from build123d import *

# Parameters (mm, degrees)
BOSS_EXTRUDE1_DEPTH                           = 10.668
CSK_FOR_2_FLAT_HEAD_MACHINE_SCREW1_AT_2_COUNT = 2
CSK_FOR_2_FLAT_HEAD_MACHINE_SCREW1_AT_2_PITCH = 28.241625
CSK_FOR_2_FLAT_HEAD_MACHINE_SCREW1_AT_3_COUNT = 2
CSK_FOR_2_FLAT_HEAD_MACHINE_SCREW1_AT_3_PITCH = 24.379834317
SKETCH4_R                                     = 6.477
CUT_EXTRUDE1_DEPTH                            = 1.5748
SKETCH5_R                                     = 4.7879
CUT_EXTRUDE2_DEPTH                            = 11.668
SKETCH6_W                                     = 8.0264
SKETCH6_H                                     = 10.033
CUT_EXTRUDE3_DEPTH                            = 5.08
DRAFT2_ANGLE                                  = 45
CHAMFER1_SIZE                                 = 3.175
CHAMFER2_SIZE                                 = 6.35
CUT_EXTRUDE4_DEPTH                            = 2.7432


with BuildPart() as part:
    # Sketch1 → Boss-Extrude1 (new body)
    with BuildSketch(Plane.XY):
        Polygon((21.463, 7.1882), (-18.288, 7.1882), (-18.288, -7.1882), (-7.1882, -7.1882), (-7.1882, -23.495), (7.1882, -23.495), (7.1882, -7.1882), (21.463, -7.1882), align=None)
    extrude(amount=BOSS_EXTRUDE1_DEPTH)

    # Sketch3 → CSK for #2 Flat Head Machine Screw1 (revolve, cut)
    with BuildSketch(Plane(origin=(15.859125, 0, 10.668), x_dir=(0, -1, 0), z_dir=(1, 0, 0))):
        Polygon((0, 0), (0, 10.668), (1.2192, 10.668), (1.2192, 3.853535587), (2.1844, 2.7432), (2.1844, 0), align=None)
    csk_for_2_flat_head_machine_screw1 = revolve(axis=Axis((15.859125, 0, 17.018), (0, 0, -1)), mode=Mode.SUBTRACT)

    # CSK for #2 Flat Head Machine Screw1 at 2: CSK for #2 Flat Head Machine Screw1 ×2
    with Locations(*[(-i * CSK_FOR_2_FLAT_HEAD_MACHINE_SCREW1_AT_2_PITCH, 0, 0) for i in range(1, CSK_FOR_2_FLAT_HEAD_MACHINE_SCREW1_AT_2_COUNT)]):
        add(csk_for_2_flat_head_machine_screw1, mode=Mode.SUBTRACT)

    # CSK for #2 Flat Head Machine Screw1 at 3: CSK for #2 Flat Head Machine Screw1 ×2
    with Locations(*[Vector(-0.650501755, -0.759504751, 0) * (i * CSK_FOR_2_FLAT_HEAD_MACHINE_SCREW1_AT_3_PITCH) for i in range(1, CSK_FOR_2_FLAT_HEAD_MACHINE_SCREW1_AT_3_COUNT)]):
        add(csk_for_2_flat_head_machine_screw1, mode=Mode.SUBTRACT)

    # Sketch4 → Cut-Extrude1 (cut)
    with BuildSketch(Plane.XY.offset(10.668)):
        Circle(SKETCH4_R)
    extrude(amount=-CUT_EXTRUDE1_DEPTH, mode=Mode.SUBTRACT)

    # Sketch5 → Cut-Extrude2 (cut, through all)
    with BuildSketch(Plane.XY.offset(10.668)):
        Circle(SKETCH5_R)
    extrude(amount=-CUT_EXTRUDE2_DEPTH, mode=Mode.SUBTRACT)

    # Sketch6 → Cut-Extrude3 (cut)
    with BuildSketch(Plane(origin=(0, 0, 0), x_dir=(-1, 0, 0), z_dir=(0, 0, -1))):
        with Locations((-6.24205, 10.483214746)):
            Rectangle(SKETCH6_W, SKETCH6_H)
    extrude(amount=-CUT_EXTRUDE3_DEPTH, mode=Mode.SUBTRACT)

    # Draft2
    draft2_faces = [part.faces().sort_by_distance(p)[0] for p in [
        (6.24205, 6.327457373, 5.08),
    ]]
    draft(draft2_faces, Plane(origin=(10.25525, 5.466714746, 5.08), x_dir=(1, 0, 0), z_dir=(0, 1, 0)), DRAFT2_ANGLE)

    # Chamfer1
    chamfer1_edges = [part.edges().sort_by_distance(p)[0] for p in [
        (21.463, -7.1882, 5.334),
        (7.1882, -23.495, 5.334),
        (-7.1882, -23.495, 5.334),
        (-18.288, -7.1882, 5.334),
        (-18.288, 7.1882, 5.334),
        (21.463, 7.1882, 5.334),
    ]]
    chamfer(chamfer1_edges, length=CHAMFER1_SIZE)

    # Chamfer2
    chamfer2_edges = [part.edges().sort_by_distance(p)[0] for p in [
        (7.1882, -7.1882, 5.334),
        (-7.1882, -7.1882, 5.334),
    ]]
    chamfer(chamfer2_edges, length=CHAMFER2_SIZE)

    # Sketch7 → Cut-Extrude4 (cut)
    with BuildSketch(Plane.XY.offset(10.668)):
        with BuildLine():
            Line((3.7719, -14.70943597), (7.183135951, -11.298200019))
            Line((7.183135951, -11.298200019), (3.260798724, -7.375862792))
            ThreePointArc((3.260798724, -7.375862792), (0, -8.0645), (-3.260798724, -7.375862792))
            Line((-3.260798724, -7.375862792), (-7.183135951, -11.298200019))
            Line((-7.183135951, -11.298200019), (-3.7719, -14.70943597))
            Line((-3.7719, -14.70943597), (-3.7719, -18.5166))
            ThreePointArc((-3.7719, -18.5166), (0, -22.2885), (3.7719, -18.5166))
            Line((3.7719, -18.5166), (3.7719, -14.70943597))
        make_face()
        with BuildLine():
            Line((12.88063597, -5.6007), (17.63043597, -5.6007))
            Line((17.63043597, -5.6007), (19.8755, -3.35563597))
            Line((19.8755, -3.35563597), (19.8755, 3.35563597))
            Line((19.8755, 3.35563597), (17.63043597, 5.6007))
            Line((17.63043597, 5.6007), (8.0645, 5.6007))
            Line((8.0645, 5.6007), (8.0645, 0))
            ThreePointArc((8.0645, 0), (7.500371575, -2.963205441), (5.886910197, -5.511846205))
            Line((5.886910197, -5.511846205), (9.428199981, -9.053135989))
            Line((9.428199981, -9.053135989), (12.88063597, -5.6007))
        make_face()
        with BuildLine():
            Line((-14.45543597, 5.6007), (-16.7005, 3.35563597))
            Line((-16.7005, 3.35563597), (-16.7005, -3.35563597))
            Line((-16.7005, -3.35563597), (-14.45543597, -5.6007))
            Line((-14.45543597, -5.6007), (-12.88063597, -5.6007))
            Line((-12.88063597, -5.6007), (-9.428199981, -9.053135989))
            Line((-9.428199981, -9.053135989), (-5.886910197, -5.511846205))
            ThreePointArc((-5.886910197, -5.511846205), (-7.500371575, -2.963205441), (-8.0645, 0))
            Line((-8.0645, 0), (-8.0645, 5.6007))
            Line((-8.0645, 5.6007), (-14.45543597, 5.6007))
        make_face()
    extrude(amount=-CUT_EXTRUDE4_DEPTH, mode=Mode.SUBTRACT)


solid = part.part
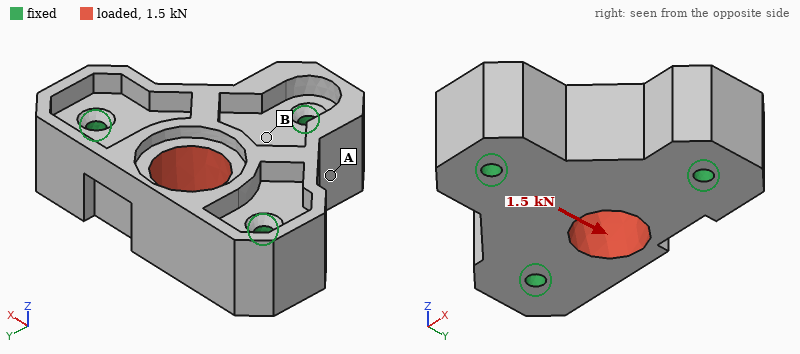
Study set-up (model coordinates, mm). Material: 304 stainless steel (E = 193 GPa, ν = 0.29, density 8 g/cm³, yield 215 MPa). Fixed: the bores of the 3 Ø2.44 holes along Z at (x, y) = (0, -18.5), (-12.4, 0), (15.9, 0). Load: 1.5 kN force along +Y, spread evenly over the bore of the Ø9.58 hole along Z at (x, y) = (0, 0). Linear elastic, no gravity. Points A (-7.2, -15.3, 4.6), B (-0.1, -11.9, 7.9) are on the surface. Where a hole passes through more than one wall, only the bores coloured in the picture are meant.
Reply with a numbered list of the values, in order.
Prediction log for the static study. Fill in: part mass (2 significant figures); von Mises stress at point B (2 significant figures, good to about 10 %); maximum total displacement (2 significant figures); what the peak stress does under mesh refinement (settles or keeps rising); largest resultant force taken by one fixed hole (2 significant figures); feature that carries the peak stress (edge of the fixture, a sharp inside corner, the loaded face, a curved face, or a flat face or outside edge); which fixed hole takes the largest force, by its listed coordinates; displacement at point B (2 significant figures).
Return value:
1. 53 g
2. 11 MPa
3. 2.0 µm
4. keeps rising
5. 690 N
6. edge of the fixture
7. (0, -18.5)
8. 0.37 µm
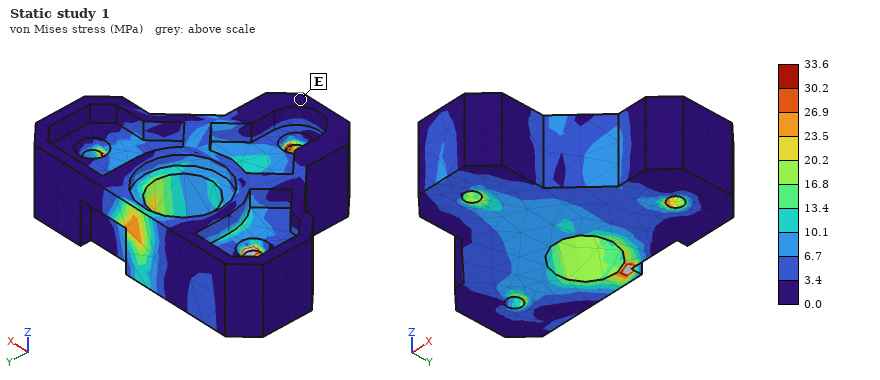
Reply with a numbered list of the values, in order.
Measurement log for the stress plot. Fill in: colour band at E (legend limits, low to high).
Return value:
1. 0.0 to 3.4 MPa
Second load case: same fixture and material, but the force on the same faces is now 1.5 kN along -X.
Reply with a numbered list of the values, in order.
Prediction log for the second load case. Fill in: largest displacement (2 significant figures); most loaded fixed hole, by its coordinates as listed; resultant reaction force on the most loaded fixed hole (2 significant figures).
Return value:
1. 0.70 µm
2. (-12.4, 0)
3. 750 N
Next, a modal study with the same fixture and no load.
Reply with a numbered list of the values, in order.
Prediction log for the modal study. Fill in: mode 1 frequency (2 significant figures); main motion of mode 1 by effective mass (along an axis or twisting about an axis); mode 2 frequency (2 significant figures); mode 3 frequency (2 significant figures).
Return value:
1. 31 kHz
2. along Z
3. 39 kHz
4. 40 kHz
